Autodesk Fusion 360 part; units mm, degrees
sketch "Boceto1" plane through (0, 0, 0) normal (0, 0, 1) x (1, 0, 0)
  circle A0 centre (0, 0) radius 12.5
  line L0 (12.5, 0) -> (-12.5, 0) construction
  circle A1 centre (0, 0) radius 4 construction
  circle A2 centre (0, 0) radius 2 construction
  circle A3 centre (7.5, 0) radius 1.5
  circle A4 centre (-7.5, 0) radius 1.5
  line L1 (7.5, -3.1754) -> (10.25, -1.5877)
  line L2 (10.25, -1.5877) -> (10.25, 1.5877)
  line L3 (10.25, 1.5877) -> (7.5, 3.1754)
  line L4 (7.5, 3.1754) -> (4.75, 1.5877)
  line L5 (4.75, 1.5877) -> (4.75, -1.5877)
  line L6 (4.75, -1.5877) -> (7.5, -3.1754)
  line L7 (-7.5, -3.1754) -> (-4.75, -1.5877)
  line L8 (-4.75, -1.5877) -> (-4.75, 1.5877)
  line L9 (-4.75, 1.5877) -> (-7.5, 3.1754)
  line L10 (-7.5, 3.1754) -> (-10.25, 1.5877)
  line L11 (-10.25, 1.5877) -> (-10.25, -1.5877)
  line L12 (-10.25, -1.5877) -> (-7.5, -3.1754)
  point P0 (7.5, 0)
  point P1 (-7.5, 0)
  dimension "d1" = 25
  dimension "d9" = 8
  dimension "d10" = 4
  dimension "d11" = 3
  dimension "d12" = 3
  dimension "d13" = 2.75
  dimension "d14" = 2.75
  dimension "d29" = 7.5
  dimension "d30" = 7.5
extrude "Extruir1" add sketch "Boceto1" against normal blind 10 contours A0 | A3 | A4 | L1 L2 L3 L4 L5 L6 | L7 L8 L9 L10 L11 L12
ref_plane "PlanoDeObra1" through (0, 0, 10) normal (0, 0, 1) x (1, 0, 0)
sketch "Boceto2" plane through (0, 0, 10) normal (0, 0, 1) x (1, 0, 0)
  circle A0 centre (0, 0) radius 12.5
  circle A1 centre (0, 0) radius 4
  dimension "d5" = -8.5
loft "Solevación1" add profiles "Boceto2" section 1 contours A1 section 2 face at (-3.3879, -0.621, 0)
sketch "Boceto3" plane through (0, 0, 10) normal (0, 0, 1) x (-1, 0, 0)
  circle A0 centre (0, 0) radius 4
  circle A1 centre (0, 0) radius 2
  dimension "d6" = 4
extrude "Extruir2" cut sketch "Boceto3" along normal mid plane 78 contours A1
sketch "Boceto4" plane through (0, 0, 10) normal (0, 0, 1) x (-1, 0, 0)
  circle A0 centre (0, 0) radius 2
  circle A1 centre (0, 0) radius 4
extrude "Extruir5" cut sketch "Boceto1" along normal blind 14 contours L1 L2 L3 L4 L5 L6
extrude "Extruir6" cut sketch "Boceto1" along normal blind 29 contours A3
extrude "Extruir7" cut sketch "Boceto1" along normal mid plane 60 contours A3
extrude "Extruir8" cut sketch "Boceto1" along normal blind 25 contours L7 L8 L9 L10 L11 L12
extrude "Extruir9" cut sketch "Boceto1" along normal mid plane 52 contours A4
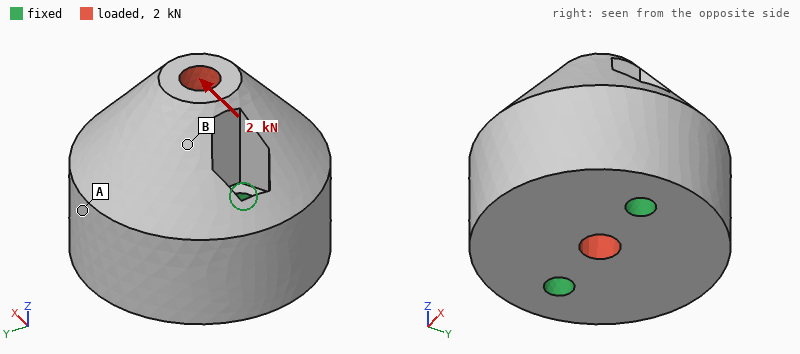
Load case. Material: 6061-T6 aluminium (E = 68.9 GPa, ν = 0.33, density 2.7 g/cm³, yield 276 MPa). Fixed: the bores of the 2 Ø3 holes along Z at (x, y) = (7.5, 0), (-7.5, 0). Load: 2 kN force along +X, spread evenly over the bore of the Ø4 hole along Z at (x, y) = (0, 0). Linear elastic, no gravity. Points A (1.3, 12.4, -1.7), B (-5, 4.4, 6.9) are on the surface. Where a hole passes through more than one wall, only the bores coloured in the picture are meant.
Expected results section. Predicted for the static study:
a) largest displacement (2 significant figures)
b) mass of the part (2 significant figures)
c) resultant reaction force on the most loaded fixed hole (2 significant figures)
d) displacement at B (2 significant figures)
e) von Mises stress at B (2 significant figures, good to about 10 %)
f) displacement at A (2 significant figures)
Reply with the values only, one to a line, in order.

4.3 µm
18 g
1.1 kN
2.7 µm
7.6 MPa
0.65 µm
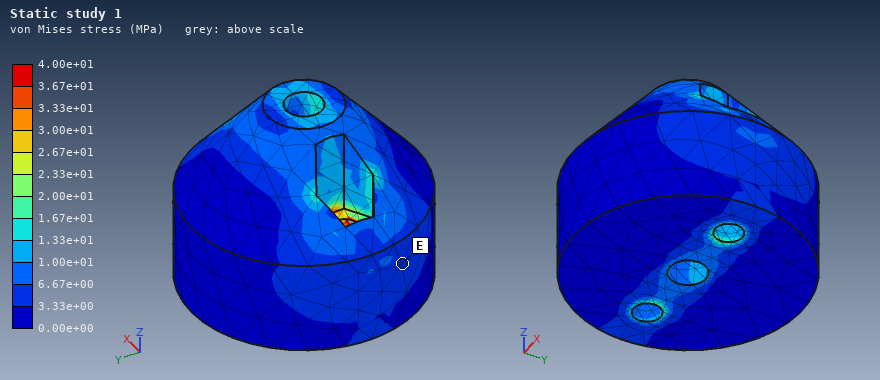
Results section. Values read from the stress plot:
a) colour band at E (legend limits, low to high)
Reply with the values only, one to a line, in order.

3.33e+00 to 6.67e+00 MPa
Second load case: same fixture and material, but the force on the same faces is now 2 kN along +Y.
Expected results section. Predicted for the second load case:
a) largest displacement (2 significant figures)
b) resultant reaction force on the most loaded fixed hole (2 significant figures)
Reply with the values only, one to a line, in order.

7.0 µm
1.0 kN
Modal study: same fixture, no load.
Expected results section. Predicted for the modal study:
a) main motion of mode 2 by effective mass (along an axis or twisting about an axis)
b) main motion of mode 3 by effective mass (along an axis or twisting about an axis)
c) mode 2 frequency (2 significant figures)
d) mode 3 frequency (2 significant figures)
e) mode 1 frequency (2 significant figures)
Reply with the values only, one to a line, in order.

along Z
along X
46 kHz
49 kHz
28 kHz
